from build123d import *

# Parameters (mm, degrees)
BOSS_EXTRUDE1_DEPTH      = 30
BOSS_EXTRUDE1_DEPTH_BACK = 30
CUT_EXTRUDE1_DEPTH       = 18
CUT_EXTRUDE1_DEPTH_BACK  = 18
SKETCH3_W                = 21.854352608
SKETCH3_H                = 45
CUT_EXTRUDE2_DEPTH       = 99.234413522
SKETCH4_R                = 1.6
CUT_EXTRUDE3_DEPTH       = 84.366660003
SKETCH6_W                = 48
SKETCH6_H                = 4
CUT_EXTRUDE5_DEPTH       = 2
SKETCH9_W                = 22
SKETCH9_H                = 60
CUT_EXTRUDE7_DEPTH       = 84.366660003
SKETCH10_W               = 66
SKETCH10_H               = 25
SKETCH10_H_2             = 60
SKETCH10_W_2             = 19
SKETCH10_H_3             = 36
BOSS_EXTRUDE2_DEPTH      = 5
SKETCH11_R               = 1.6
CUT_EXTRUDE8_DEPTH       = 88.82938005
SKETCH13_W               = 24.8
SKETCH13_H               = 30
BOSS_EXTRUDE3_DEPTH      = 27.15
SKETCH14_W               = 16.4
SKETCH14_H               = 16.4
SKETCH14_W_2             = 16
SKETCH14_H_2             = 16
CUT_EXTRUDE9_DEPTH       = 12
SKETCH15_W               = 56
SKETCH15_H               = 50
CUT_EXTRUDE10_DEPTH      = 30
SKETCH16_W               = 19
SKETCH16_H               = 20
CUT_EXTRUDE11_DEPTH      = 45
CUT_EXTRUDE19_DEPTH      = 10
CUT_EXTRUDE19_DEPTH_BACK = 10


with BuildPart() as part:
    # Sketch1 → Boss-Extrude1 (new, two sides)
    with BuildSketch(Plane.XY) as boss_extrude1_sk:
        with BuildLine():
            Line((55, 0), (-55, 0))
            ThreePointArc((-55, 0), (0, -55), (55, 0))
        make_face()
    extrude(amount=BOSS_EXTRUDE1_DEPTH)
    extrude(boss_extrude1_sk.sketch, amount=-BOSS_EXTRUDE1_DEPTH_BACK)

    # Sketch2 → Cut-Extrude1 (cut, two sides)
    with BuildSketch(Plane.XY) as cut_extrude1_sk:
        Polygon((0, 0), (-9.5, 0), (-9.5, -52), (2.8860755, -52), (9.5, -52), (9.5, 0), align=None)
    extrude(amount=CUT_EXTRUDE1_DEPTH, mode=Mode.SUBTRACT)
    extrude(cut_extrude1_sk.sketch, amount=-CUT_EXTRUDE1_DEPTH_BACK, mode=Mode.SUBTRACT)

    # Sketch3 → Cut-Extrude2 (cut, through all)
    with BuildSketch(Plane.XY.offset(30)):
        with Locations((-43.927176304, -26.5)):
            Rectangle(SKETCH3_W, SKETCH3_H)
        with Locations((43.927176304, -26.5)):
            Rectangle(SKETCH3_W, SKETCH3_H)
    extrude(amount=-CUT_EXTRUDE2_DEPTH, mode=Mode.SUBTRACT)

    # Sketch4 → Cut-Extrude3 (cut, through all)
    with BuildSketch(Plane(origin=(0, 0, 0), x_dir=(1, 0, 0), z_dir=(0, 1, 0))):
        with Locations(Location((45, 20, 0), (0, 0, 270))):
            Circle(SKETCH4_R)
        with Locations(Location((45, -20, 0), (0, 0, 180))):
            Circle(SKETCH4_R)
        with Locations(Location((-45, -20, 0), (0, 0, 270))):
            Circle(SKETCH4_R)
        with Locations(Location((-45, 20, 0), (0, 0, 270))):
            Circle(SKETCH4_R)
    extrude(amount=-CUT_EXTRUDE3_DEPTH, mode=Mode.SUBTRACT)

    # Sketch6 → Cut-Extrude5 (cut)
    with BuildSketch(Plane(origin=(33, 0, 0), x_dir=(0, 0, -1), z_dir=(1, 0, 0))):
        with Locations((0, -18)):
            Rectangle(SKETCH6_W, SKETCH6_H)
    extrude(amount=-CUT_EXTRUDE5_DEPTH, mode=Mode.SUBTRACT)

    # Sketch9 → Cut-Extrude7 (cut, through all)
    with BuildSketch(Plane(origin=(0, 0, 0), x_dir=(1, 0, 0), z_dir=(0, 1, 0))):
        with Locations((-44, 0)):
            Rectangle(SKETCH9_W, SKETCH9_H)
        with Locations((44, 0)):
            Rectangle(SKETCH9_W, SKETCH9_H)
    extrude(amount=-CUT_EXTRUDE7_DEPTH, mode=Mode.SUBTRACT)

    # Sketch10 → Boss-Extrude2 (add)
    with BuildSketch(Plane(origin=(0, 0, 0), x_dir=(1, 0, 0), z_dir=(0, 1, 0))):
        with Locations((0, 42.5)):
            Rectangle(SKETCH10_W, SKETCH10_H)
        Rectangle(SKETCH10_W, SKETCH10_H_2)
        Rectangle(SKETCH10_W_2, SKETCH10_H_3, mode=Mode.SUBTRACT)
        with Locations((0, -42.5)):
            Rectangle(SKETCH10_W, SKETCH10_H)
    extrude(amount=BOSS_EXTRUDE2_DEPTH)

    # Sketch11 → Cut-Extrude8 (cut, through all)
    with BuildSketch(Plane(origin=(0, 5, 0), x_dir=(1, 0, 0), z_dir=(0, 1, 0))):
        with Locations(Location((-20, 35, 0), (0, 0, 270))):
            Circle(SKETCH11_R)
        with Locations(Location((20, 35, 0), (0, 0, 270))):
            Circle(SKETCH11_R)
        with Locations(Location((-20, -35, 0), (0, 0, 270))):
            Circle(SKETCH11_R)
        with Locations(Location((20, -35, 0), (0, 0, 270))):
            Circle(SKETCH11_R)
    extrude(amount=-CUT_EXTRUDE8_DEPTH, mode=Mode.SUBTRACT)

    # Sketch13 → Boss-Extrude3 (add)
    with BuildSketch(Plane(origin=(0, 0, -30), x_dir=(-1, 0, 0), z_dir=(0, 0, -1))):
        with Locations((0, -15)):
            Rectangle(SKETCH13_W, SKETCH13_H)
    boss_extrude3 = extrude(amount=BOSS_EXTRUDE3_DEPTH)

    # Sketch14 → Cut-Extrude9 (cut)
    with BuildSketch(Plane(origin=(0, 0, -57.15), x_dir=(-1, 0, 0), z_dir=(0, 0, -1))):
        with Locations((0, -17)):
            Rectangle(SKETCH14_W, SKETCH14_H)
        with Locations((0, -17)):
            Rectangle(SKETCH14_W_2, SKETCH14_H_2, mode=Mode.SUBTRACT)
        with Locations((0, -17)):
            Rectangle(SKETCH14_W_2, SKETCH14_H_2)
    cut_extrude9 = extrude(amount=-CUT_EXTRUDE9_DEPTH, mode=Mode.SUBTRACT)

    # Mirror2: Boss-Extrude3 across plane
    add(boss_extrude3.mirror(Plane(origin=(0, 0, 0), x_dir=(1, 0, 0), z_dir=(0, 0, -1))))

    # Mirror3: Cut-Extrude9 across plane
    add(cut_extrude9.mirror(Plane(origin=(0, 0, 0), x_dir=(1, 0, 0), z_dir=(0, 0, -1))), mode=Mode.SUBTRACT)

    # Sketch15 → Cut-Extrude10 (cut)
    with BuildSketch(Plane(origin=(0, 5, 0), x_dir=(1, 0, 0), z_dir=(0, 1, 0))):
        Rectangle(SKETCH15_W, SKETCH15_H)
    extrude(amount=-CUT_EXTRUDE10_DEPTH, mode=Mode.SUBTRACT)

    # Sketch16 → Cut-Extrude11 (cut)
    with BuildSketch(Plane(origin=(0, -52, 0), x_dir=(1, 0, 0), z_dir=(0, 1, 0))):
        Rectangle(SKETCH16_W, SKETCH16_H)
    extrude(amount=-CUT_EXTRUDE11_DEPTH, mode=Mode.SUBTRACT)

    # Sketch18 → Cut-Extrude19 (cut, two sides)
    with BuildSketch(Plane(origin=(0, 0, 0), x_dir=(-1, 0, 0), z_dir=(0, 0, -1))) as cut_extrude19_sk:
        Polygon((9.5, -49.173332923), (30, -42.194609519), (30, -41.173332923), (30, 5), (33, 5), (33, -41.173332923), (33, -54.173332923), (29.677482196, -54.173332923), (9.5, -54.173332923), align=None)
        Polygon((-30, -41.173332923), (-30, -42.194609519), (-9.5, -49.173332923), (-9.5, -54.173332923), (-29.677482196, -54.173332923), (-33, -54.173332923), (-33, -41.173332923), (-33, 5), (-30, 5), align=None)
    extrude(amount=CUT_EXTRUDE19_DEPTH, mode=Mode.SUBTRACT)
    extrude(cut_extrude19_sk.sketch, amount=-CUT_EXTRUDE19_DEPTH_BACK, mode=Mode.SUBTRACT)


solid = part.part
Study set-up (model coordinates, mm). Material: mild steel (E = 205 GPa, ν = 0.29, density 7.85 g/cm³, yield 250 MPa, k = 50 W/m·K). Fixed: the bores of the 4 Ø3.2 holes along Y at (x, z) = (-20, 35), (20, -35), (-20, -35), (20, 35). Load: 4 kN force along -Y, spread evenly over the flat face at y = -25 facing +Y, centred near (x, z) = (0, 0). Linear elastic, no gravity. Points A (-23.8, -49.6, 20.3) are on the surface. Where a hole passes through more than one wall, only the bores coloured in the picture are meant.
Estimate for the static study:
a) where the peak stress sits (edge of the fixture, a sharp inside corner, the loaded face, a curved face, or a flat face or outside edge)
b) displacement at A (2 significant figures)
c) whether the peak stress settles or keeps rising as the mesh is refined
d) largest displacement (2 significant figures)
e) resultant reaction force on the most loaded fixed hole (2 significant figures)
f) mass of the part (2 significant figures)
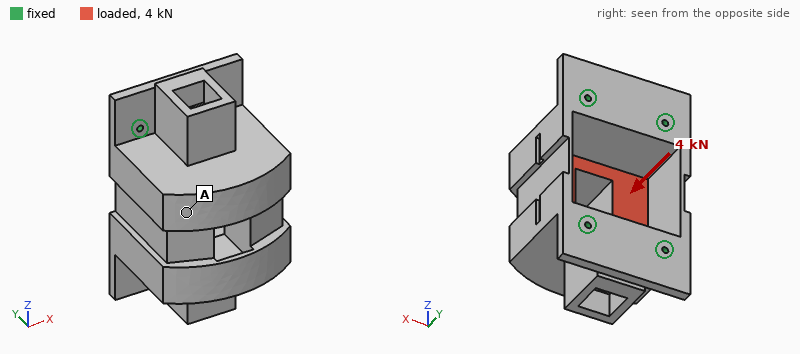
edge of the fixture
2.6 µm
keeps rising
3.4 µm
1.1 kN
1.3 kg
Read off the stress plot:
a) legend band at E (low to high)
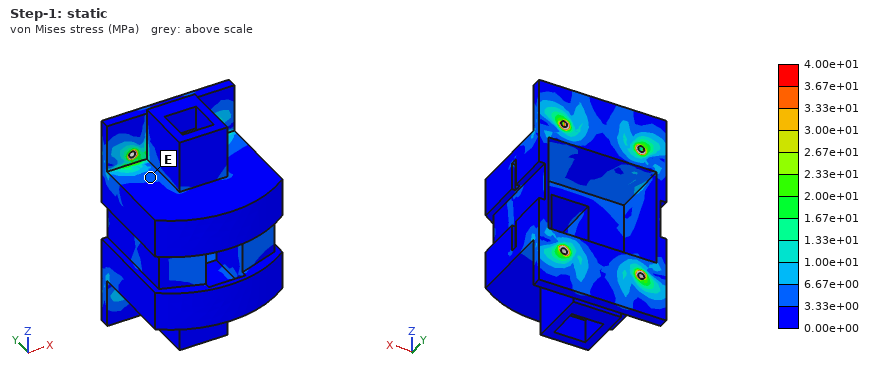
3.33e+00 to 6.67e+00 MPa
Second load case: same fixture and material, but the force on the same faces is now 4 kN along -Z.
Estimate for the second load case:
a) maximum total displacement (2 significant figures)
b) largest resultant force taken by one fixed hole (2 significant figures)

8.1 µm
1.3 kN
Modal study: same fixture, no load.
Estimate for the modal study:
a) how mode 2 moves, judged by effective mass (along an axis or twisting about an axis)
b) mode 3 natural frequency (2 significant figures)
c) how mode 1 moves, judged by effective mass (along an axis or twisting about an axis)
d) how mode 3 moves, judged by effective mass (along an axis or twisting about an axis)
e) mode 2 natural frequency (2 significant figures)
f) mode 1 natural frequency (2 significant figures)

along Z
6100 Hz
along X
along Y
4000 Hz
3200 Hz
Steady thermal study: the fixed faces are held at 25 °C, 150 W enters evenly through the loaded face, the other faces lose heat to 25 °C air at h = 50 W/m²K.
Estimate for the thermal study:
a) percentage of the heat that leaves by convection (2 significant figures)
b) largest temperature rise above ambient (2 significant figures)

56 %
80 K
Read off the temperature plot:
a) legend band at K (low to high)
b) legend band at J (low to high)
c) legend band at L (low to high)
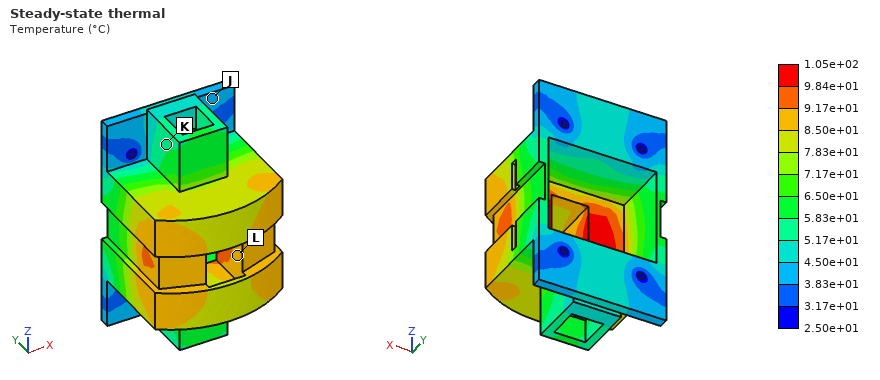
5.17e+01 to 5.83e+01 °C
3.83e+01 to 4.50e+01 °C
8.50e+01 to 9.17e+01 °C
